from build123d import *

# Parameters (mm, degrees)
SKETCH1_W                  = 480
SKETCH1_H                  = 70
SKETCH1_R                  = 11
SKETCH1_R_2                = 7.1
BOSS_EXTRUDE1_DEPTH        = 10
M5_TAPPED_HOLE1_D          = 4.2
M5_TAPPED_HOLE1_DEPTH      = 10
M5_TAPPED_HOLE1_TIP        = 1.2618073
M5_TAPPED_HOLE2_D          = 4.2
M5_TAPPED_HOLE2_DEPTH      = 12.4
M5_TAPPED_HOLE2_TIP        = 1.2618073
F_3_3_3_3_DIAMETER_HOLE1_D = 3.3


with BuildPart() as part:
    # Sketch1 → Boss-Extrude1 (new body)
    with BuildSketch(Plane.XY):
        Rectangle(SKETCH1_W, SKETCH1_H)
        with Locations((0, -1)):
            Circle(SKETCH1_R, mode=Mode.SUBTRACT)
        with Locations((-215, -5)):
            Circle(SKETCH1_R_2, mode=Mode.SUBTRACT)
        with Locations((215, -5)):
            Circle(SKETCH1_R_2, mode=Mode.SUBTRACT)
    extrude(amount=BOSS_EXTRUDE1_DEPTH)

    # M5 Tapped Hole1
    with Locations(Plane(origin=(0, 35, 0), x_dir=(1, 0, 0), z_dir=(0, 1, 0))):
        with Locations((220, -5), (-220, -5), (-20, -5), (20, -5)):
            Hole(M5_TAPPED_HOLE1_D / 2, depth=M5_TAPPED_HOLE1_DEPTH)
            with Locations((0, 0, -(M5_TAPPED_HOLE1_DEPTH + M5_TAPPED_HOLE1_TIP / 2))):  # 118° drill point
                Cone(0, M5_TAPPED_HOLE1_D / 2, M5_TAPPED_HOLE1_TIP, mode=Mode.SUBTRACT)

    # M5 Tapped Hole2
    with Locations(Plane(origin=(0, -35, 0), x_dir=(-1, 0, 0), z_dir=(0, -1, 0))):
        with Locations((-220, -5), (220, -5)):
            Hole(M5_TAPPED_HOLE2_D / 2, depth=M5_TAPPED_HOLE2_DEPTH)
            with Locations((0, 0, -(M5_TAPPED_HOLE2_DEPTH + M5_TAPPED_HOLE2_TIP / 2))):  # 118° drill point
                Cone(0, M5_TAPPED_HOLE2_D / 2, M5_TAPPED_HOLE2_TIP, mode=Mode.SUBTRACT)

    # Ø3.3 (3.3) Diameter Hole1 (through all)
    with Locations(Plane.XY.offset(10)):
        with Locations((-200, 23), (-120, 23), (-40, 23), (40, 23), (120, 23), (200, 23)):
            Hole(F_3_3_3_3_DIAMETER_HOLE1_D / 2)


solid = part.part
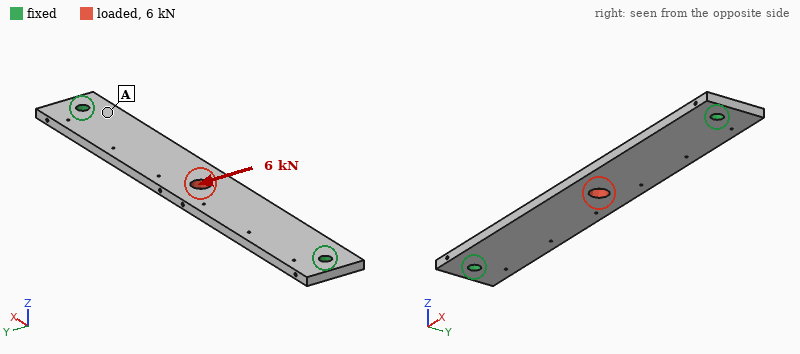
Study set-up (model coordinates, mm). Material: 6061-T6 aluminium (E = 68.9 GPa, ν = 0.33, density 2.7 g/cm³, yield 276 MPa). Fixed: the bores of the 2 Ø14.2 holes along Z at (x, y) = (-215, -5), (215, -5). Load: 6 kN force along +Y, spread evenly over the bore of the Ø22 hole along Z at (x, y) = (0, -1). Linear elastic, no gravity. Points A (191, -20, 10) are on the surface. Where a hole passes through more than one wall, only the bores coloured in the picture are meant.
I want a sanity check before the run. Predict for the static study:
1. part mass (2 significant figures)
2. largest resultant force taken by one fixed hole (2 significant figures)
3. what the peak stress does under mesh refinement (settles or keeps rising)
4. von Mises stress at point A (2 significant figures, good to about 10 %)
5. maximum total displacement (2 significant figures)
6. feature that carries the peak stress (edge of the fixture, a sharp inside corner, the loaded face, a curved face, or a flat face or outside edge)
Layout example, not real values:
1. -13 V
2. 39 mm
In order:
1. 880 g
2. 3.3 kN
3. keeps rising
4. 15 MPa
5. 0.29 mm
6. edge of the fixture
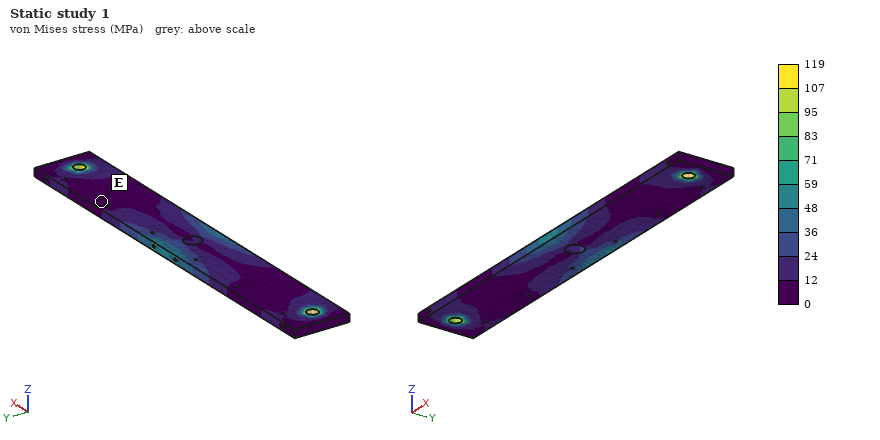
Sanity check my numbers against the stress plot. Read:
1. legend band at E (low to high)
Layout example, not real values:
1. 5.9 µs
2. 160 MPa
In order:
1. 0 to 12 MPa
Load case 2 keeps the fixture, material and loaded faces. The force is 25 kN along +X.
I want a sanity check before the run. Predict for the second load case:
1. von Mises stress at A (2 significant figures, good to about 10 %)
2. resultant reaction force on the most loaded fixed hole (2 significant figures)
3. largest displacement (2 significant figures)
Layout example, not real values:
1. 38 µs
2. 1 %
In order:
1. 22 MPa
2. 13 kN
3. 66 µm
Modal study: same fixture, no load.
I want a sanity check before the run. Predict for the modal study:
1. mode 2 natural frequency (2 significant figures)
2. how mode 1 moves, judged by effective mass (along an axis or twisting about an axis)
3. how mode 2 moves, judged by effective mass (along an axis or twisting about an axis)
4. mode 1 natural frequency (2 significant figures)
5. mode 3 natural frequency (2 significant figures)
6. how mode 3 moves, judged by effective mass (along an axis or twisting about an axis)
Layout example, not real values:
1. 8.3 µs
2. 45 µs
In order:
1. 780 Hz
2. along Z
3. twisting about Y
4. 280 Hz
5. 1000 Hz
6. twisting about X
